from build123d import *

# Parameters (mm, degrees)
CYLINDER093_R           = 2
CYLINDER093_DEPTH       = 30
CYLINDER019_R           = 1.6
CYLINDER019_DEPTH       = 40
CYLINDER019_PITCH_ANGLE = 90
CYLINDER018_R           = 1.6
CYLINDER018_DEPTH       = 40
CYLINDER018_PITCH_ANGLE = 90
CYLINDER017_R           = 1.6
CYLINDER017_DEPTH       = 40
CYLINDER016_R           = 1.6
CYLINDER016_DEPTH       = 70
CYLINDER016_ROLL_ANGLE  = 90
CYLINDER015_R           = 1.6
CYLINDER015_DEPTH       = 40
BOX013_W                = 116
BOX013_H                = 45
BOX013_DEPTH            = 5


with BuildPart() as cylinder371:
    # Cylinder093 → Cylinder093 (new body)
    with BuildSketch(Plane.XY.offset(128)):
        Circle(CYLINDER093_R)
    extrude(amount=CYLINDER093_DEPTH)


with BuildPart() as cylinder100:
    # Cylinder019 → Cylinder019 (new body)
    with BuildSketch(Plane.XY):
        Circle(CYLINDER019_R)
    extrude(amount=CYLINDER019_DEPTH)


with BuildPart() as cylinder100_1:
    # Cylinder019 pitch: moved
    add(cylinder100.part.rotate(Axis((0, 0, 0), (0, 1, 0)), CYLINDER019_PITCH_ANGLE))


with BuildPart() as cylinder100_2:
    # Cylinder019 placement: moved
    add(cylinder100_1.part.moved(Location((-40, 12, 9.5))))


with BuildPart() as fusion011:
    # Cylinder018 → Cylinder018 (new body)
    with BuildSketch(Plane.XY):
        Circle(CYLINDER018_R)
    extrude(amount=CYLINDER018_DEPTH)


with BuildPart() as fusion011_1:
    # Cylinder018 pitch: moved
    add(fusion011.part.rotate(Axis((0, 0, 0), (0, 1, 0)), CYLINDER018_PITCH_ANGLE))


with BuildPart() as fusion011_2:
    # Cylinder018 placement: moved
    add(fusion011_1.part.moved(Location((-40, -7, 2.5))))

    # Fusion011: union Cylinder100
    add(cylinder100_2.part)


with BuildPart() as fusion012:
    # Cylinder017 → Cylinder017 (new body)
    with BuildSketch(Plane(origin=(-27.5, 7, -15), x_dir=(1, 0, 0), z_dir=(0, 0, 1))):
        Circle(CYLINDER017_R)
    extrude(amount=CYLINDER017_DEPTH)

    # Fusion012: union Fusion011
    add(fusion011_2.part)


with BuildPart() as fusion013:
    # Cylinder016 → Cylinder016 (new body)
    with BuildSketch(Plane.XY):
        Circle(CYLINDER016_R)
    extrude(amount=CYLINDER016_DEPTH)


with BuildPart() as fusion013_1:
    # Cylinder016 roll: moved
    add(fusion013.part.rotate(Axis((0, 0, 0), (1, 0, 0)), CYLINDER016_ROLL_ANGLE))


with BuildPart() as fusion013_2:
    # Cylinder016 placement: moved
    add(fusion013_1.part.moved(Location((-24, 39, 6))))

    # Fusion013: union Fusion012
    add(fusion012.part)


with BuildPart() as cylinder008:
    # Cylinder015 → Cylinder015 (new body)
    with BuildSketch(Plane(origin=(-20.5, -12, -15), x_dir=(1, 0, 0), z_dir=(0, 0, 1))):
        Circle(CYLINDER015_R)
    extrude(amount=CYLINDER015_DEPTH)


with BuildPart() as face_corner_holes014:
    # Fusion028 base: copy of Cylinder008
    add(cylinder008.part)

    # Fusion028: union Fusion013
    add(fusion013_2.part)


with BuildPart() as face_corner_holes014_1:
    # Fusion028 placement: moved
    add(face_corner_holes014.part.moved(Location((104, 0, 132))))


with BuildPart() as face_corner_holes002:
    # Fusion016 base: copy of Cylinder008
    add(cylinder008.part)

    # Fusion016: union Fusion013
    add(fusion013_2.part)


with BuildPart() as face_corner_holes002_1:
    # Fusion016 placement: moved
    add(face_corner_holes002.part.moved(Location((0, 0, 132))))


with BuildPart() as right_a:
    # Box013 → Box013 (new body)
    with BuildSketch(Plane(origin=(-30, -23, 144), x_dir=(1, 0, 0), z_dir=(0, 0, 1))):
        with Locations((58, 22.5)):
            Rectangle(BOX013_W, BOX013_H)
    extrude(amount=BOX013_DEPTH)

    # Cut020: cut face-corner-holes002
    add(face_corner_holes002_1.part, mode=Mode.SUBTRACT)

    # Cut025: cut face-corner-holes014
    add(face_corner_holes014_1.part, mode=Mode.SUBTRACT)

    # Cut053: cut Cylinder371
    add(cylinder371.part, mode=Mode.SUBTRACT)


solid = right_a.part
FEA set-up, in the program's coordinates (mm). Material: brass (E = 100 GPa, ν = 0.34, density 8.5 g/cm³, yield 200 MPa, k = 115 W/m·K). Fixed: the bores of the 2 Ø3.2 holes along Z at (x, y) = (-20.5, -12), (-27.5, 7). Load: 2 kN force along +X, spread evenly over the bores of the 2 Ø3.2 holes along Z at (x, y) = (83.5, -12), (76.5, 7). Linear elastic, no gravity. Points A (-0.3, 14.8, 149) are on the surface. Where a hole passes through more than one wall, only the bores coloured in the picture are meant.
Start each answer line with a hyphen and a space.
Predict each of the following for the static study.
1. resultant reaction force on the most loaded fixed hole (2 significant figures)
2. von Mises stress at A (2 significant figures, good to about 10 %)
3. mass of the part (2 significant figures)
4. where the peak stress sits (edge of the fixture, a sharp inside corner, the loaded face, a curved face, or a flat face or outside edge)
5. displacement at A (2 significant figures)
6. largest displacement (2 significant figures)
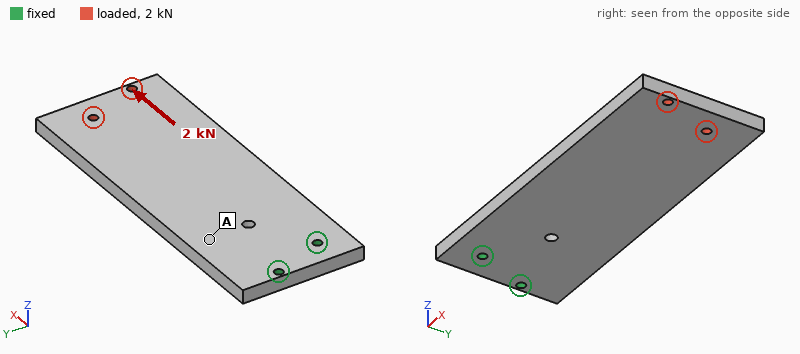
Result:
- 1.0 kN
- 7.1 MPa
- 220 g
- a flat face or outside edge
- 4.1 µm
- 14 µm
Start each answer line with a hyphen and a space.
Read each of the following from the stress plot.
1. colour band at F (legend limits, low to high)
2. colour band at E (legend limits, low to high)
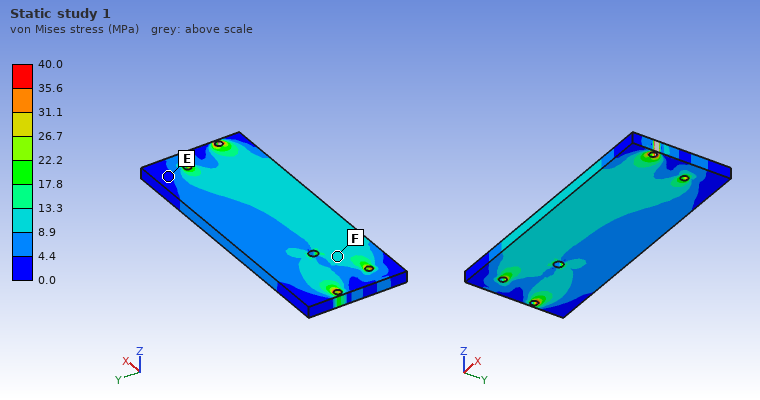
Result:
- 8.9 to 13.3 MPa
- 0.0 to 4.4 MPa
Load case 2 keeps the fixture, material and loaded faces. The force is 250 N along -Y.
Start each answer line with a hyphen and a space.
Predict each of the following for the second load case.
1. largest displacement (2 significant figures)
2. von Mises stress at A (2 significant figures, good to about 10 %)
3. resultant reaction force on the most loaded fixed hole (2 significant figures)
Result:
- 49 µm
- 8.3 MPa
- 1.2 kN
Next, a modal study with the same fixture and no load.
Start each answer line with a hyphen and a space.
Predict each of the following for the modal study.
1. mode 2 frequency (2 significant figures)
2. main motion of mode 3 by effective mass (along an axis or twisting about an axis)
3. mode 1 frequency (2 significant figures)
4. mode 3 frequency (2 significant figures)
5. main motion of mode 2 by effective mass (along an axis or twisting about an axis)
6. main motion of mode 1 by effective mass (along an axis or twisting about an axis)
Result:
- 1100 Hz
- along Y
- 230 Hz
- 1400 Hz
- twisting about X
- along Z
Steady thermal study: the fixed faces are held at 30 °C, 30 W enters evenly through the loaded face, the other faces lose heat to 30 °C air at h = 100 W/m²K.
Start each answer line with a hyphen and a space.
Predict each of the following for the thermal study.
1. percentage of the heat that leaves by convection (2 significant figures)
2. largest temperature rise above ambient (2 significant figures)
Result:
- 79 %
- 62 K
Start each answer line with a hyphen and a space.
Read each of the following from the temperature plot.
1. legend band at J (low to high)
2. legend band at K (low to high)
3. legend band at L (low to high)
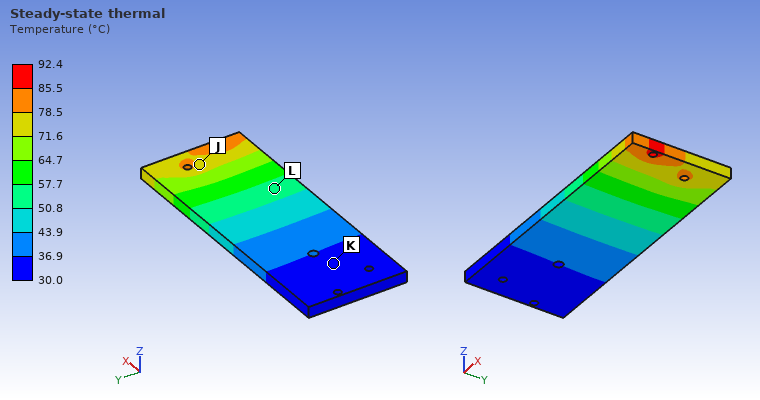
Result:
- 71.6 to 78.5 °C
- 30.0 to 36.9 °C
- 50.8 to 57.7 °C
